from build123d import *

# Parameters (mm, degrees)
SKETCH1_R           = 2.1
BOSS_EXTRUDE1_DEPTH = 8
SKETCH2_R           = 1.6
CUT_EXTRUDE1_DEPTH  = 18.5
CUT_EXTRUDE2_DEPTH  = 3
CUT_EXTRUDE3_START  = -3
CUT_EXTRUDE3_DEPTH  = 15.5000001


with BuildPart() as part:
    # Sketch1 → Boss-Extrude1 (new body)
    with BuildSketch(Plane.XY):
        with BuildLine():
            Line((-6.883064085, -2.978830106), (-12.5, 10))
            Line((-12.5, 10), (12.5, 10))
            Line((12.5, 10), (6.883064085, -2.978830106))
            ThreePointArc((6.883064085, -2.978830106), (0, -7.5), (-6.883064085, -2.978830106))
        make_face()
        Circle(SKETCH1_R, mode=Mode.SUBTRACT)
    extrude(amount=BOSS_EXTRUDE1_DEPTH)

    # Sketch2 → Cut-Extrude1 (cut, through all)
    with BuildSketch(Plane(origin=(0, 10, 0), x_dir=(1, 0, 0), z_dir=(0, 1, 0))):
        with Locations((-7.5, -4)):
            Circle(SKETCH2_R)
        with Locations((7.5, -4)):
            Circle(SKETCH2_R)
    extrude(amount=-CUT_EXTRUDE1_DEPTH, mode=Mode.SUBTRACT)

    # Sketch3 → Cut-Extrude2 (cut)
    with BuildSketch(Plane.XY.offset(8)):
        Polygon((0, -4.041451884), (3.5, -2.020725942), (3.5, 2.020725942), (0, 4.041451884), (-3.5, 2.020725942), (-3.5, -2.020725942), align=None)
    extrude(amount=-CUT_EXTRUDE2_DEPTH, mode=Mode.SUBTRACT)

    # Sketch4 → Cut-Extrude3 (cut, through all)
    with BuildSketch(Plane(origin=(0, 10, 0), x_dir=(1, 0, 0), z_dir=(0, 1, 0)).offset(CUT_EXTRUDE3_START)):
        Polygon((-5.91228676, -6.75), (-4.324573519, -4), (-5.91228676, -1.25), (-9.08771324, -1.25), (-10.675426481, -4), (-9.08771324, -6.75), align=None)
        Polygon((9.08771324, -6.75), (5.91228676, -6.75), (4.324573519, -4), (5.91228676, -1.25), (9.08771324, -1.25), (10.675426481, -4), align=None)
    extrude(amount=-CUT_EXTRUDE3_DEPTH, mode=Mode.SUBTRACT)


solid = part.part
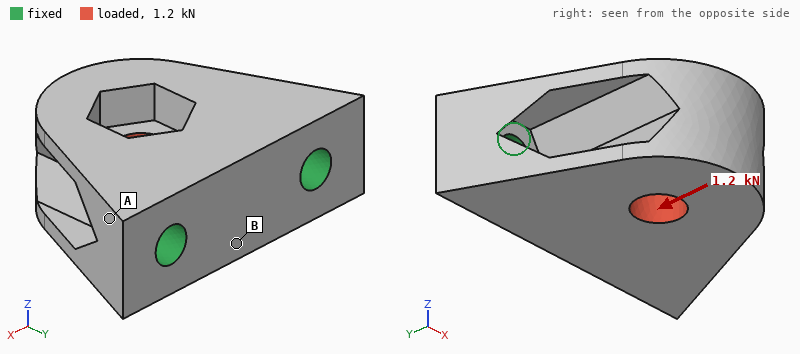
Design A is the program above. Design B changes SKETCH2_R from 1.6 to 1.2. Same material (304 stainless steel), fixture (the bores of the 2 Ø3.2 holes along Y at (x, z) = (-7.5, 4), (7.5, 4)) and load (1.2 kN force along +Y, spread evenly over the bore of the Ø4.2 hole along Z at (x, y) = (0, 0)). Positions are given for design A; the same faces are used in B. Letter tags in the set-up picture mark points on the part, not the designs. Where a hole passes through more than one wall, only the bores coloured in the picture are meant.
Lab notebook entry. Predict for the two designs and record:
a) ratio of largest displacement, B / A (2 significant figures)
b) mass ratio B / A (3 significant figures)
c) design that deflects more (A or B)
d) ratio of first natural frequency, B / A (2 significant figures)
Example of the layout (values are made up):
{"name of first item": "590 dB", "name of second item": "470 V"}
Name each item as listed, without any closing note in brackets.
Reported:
{"ratio of largest displacement, B / A": "1.3", "mass ratio B / A": "1.01", "design that deflects more": "B", "ratio of first natural frequency, B / A": "0.87"}
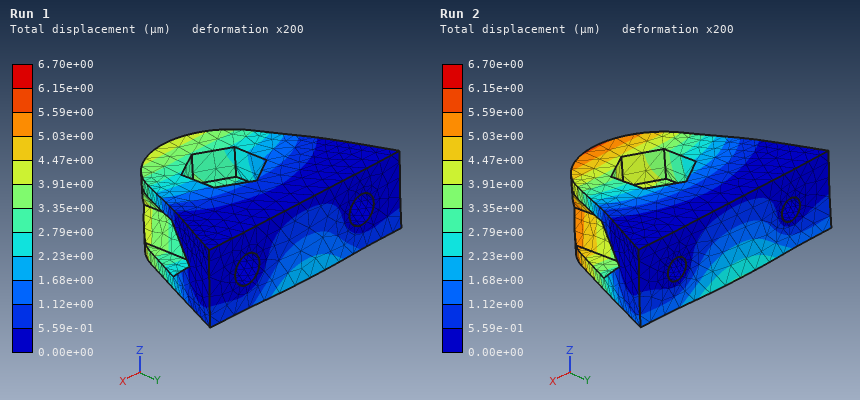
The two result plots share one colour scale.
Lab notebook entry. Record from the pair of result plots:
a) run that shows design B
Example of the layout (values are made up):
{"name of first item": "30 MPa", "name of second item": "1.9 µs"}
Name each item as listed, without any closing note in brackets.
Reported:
{"run that shows design B": "Run 2"}
